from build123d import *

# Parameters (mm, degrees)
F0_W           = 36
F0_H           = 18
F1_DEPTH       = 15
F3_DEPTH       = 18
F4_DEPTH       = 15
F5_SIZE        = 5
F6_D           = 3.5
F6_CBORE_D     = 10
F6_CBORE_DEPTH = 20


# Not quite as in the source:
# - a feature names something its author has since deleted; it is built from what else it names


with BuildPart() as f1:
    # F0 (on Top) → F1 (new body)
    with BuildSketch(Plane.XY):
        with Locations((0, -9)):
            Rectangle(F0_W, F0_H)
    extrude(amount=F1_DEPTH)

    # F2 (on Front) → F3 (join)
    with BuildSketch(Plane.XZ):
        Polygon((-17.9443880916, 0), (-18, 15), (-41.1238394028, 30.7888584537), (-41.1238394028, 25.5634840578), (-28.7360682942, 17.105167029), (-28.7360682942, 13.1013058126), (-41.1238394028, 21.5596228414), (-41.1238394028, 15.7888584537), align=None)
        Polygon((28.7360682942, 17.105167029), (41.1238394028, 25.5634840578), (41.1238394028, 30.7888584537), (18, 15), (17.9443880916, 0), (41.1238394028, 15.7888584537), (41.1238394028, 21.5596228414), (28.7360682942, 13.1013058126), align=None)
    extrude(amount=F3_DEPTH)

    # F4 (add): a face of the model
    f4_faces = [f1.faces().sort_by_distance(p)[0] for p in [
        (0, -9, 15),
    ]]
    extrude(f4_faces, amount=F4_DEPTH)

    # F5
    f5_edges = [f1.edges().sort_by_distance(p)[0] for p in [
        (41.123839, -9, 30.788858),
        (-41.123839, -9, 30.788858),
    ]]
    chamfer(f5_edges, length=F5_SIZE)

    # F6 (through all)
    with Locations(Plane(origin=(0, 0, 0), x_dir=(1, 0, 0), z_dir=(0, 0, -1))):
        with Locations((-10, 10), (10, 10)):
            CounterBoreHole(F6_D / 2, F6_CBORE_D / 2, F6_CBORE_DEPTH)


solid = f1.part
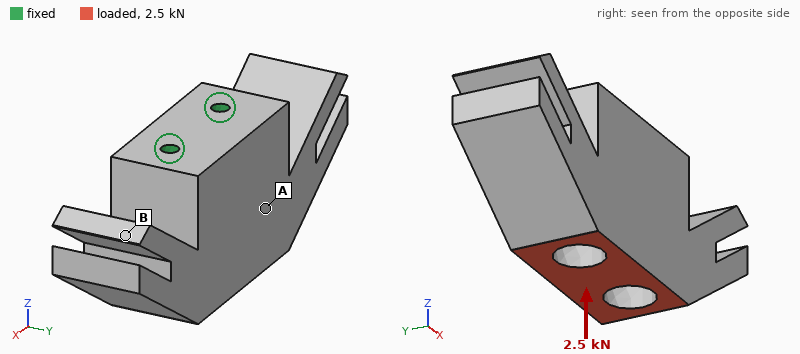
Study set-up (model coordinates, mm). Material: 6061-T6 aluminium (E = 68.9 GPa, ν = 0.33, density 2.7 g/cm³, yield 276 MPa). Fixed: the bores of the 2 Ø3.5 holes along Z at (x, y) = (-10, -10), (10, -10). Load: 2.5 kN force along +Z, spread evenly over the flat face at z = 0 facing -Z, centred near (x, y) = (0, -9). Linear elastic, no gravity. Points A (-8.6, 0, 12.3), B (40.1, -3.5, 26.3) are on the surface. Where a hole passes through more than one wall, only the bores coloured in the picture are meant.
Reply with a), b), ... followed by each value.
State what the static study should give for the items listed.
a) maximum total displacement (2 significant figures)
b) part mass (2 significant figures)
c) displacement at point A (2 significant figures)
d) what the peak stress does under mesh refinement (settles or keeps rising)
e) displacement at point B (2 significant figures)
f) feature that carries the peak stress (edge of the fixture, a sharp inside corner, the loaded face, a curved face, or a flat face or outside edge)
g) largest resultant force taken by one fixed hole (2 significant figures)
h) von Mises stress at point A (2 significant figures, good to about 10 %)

a) 4.5 µm
b) 71 g
c) 3.2 µm
d) keeps rising
e) 3.0 µm
f) edge of the fixture
g) 1.3 kN
h) 5.4 MPa
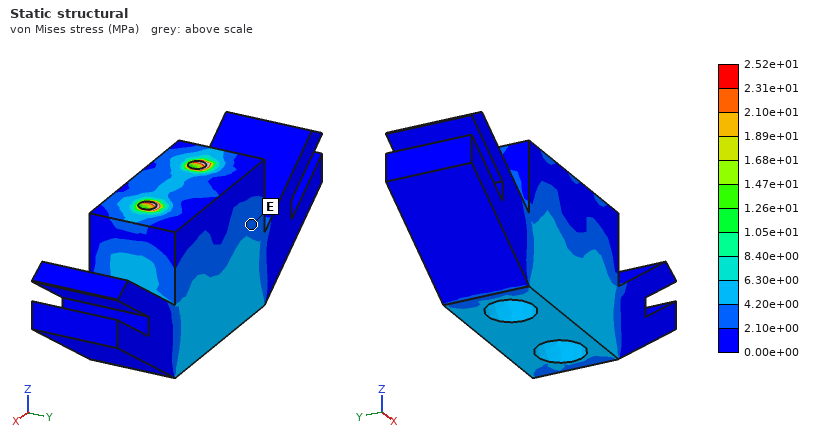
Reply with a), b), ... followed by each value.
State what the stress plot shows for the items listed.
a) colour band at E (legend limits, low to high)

a) 2.10e+00 to 4.20e+00 MPa
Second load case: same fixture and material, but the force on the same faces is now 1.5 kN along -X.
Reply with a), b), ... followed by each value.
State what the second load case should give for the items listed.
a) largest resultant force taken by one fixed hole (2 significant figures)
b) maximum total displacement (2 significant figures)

a) 1.6 kN
b) 15 µm
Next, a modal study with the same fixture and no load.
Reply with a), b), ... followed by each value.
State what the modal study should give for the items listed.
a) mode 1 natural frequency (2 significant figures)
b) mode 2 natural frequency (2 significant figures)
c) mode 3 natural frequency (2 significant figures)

a) 7300 Hz
b) 7500 Hz
c) 7700 Hz
